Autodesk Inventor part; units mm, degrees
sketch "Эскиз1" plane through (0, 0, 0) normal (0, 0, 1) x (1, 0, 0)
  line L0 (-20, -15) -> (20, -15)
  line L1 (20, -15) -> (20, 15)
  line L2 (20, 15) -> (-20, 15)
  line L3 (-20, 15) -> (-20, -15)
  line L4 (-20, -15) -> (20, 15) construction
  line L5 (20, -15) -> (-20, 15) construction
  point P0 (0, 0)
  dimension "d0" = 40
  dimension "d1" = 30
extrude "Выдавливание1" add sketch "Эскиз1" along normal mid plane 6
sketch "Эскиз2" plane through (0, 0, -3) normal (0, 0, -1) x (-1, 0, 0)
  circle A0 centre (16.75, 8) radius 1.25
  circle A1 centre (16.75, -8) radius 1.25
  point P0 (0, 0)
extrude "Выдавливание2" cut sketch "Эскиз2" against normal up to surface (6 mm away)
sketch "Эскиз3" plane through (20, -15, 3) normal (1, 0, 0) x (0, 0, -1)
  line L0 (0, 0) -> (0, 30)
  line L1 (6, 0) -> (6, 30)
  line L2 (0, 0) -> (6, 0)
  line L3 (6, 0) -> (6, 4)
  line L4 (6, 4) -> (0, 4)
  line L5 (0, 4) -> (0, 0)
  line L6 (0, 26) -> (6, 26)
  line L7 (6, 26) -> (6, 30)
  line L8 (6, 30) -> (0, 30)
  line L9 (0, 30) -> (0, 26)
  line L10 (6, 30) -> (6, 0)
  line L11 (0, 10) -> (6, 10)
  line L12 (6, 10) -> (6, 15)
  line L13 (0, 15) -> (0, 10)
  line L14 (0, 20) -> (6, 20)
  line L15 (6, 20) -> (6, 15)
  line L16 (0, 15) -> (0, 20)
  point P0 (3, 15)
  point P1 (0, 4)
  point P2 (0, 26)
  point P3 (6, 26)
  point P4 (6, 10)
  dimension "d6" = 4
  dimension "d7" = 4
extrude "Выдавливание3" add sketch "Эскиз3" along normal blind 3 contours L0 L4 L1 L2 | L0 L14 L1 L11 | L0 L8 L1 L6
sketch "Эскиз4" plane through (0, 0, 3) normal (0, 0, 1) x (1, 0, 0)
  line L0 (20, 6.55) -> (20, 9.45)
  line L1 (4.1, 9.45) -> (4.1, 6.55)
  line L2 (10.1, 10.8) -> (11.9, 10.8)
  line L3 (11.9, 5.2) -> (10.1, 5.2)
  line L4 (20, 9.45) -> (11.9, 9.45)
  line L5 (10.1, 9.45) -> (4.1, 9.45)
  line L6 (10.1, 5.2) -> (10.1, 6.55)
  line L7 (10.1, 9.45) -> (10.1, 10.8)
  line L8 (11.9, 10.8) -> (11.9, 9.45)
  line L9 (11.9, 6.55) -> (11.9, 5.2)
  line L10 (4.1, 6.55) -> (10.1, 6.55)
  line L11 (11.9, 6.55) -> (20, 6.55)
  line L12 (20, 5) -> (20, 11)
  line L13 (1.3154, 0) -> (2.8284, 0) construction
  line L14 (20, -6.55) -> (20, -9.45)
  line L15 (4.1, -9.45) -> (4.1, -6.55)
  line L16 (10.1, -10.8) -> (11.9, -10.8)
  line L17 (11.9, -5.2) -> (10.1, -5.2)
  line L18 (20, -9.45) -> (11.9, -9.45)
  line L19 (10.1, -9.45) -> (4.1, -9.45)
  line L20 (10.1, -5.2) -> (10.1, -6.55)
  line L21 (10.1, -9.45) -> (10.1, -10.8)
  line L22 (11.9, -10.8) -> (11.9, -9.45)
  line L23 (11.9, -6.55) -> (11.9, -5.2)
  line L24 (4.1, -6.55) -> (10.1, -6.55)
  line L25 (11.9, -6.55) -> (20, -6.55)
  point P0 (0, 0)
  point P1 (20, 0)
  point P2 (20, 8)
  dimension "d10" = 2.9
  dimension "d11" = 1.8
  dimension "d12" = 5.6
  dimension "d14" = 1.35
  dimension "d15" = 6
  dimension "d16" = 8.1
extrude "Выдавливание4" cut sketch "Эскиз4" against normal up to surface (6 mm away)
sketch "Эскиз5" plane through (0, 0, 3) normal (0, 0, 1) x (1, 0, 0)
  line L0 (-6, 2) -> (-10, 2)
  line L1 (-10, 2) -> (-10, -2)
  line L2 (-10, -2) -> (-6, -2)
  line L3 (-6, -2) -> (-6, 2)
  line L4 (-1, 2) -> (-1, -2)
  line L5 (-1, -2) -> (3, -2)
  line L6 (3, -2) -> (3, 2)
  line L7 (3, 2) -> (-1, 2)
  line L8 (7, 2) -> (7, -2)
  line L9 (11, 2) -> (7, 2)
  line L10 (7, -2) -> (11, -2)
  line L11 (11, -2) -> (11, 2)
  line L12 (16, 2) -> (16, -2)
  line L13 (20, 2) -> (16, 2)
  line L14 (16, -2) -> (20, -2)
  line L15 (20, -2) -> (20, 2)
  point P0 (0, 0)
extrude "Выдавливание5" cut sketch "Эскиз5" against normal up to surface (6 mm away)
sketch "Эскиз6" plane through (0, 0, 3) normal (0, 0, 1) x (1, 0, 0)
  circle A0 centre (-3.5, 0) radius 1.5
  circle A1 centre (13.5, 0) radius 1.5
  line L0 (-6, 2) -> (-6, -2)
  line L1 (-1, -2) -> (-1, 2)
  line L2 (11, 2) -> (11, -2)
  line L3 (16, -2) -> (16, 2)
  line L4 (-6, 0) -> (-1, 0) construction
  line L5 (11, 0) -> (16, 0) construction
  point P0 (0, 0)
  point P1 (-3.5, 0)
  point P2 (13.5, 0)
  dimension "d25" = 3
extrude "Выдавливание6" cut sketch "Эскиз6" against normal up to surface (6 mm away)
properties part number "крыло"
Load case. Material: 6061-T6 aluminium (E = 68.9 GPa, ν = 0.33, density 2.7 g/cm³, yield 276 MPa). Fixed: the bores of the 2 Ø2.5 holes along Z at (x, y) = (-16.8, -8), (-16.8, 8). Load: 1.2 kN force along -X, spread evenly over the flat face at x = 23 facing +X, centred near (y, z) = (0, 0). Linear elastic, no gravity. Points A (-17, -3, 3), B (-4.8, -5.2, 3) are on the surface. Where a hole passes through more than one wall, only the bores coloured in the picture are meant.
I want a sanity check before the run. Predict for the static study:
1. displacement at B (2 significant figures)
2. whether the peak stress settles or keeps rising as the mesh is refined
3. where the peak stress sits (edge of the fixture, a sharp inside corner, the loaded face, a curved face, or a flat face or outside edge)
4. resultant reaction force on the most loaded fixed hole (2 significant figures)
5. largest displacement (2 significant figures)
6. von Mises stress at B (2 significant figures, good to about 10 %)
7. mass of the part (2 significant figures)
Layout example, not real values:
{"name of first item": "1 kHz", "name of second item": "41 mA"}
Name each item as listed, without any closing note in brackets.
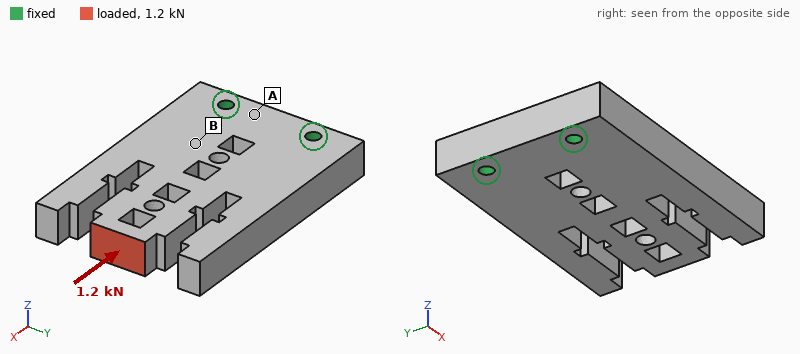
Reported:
{"displacement at B": "2.1 µm", "whether the peak stress settles or keeps rising as the mesh is refined": "keeps rising", "where the peak stress sits": "a sharp inside corner", "resultant reaction force on the most loaded fixed hole": "610 N", "largest displacement": "13 µm", "von Mises stress at B": "13 MPa", "mass of the part": "17 g"}
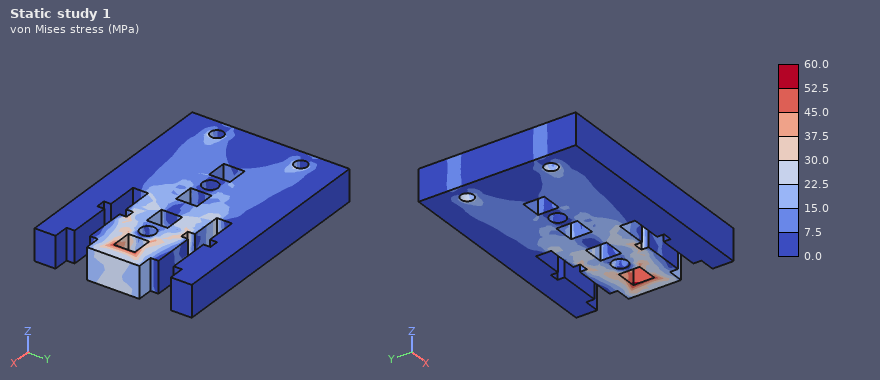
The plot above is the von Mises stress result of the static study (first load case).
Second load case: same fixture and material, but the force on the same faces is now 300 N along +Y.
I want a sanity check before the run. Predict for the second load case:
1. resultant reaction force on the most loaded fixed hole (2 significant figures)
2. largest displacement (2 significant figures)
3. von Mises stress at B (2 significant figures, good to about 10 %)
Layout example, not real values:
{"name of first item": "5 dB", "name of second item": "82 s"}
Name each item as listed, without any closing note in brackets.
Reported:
{"resultant reaction force on the most loaded fixed hole": "690 N", "largest displacement": "43 µm", "von Mises stress at B": "9.2 MPa"}
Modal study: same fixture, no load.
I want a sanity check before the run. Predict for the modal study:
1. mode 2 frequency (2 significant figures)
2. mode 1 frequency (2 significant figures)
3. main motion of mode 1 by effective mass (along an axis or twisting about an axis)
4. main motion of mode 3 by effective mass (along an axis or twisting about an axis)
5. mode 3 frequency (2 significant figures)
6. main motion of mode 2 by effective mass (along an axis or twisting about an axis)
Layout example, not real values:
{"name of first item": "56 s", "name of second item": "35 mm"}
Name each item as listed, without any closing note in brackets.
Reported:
{"mode 2 frequency": "5800 Hz", "mode 1 frequency": "3300 Hz", "main motion of mode 1 by effective mass": "along Z", "main motion of mode 3 by effective mass": "along Y", "mode 3 frequency": "7400 Hz", "main motion of mode 2 by effective mass": "twisting about X"}
